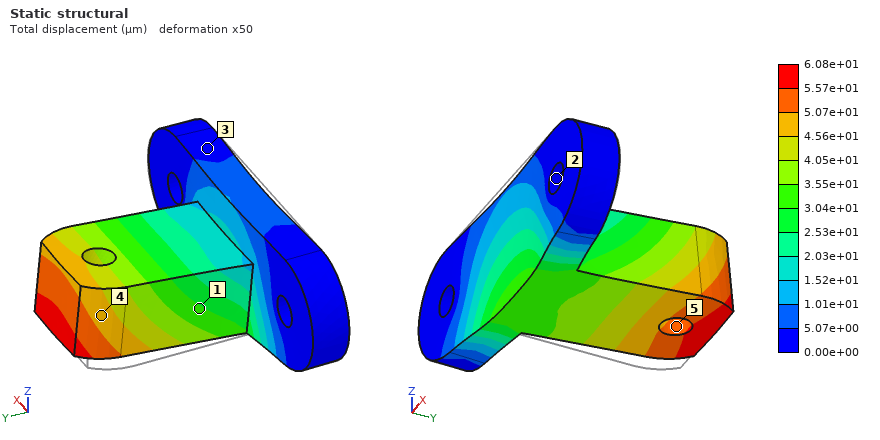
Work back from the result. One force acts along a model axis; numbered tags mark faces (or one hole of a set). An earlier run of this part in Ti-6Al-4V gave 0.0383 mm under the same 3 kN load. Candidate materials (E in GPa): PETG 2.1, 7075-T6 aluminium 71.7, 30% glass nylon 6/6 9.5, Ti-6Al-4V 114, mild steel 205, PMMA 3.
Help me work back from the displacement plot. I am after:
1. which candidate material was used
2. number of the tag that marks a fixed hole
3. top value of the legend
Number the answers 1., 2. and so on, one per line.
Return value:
1. 7075-T6 aluminium
2. 2
3. 6.08e+01 µm
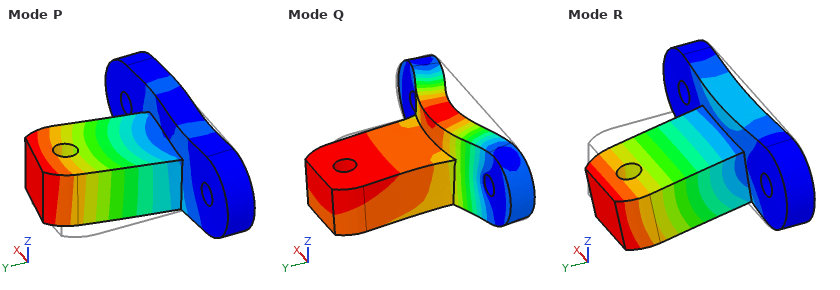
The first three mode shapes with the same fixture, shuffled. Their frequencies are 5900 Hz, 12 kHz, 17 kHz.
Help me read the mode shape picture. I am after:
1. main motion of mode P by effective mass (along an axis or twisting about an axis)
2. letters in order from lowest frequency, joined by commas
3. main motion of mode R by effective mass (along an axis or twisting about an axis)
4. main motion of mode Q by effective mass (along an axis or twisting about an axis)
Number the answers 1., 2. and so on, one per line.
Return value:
1. along X
2. R, P, Q
3. along Z
4. along Y
